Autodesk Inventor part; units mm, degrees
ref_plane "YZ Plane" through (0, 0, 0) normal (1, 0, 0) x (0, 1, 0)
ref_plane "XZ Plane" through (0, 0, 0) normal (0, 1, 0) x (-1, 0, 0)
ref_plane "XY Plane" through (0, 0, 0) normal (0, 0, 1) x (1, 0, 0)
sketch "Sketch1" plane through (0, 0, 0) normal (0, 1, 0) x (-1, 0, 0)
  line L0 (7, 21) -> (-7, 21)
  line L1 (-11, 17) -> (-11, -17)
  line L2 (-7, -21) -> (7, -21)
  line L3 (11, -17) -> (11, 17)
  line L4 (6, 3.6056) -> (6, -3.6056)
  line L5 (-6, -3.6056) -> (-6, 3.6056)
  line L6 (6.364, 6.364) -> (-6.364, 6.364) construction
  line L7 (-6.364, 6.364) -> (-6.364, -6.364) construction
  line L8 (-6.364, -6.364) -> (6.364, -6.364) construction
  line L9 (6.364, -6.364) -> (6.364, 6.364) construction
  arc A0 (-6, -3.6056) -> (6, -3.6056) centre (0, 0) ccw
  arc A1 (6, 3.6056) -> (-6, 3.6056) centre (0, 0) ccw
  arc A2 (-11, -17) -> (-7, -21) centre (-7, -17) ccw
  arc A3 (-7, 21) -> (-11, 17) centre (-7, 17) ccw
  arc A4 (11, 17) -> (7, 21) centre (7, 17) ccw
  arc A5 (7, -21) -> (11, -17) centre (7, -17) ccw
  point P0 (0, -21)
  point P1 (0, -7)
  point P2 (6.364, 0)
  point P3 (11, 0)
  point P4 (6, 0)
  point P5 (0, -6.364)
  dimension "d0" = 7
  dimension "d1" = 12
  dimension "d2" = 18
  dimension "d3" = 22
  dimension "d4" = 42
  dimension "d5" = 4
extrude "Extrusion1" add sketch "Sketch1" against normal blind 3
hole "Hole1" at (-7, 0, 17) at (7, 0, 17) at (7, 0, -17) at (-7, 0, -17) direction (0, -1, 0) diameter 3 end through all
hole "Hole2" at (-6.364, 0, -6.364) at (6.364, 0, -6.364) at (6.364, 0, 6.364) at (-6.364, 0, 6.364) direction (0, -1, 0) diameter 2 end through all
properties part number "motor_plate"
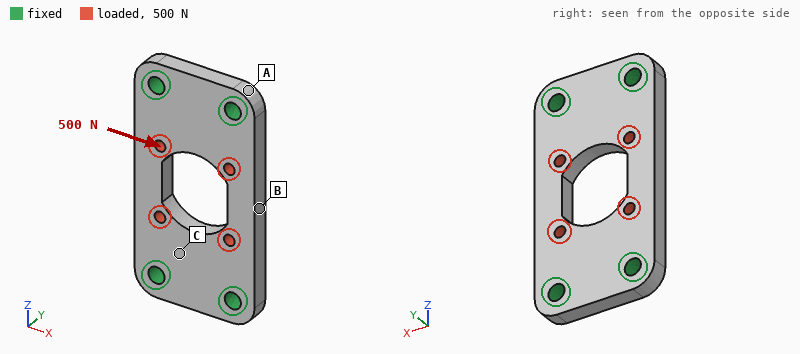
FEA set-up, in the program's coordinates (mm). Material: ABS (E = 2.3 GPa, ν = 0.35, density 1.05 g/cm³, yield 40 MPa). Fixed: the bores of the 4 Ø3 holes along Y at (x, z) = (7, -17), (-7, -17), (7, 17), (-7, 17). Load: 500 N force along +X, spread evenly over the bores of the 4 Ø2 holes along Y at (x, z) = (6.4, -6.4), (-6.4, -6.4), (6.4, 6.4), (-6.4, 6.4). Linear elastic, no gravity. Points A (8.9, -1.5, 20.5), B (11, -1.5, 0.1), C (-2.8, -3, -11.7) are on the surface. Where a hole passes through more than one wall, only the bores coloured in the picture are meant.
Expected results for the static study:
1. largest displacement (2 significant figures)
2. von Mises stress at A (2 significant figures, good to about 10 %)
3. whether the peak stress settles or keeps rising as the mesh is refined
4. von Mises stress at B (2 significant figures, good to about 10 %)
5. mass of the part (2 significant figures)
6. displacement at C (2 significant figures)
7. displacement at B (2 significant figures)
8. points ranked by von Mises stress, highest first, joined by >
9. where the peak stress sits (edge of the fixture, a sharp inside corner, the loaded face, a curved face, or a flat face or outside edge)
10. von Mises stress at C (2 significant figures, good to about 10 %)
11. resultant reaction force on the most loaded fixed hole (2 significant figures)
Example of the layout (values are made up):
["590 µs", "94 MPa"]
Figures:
["87 µm", "2.5 MPa", "keeps rising", "6.1 MPa", "2.3 g", "30 µm", "84 µm", "C > B > A", "edge of the fixture", "9.3 MPa", "160 N"]
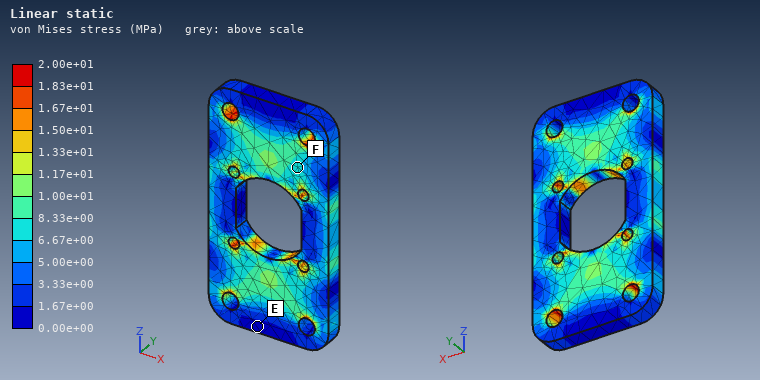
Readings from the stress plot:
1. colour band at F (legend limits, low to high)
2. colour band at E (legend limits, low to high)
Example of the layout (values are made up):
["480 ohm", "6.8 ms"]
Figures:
["6.67e+00 to 8.33e+00 MPa", "0.00e+00 to 1.67e+00 MPa"]
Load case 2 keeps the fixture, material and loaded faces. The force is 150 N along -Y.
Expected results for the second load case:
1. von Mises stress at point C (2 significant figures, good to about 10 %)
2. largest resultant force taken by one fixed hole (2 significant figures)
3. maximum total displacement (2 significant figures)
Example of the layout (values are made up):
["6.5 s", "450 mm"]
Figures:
["6.4 MPa", "38 N", "0.25 mm"]
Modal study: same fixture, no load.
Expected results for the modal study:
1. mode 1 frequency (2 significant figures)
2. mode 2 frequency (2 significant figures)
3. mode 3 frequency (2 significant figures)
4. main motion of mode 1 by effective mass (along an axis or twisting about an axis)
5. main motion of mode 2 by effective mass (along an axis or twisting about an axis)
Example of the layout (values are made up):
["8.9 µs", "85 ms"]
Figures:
["4500 Hz", "5300 Hz", "9100 Hz", "along Y", "twisting about Z"]
